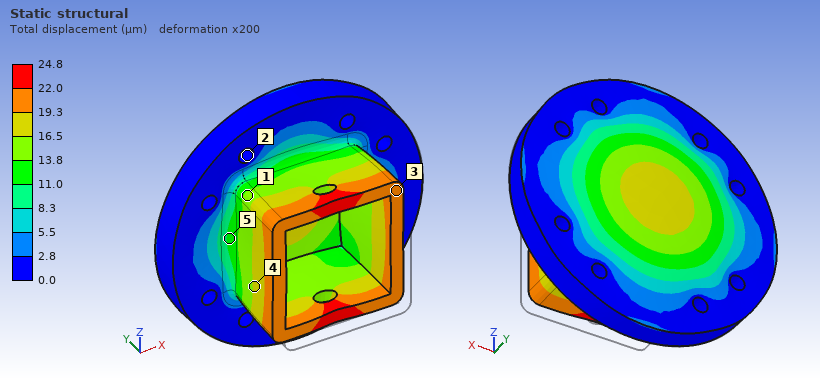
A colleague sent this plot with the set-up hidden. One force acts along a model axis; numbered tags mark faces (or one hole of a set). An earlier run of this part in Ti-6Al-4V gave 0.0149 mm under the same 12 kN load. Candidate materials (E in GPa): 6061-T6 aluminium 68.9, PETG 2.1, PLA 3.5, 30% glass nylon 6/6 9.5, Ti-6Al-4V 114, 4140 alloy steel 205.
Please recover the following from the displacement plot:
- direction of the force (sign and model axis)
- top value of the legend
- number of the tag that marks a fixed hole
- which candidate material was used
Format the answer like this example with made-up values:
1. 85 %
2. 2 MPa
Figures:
1. +Y
2. 24.8 µm
3. 2
4. 6061-T6 aluminium
